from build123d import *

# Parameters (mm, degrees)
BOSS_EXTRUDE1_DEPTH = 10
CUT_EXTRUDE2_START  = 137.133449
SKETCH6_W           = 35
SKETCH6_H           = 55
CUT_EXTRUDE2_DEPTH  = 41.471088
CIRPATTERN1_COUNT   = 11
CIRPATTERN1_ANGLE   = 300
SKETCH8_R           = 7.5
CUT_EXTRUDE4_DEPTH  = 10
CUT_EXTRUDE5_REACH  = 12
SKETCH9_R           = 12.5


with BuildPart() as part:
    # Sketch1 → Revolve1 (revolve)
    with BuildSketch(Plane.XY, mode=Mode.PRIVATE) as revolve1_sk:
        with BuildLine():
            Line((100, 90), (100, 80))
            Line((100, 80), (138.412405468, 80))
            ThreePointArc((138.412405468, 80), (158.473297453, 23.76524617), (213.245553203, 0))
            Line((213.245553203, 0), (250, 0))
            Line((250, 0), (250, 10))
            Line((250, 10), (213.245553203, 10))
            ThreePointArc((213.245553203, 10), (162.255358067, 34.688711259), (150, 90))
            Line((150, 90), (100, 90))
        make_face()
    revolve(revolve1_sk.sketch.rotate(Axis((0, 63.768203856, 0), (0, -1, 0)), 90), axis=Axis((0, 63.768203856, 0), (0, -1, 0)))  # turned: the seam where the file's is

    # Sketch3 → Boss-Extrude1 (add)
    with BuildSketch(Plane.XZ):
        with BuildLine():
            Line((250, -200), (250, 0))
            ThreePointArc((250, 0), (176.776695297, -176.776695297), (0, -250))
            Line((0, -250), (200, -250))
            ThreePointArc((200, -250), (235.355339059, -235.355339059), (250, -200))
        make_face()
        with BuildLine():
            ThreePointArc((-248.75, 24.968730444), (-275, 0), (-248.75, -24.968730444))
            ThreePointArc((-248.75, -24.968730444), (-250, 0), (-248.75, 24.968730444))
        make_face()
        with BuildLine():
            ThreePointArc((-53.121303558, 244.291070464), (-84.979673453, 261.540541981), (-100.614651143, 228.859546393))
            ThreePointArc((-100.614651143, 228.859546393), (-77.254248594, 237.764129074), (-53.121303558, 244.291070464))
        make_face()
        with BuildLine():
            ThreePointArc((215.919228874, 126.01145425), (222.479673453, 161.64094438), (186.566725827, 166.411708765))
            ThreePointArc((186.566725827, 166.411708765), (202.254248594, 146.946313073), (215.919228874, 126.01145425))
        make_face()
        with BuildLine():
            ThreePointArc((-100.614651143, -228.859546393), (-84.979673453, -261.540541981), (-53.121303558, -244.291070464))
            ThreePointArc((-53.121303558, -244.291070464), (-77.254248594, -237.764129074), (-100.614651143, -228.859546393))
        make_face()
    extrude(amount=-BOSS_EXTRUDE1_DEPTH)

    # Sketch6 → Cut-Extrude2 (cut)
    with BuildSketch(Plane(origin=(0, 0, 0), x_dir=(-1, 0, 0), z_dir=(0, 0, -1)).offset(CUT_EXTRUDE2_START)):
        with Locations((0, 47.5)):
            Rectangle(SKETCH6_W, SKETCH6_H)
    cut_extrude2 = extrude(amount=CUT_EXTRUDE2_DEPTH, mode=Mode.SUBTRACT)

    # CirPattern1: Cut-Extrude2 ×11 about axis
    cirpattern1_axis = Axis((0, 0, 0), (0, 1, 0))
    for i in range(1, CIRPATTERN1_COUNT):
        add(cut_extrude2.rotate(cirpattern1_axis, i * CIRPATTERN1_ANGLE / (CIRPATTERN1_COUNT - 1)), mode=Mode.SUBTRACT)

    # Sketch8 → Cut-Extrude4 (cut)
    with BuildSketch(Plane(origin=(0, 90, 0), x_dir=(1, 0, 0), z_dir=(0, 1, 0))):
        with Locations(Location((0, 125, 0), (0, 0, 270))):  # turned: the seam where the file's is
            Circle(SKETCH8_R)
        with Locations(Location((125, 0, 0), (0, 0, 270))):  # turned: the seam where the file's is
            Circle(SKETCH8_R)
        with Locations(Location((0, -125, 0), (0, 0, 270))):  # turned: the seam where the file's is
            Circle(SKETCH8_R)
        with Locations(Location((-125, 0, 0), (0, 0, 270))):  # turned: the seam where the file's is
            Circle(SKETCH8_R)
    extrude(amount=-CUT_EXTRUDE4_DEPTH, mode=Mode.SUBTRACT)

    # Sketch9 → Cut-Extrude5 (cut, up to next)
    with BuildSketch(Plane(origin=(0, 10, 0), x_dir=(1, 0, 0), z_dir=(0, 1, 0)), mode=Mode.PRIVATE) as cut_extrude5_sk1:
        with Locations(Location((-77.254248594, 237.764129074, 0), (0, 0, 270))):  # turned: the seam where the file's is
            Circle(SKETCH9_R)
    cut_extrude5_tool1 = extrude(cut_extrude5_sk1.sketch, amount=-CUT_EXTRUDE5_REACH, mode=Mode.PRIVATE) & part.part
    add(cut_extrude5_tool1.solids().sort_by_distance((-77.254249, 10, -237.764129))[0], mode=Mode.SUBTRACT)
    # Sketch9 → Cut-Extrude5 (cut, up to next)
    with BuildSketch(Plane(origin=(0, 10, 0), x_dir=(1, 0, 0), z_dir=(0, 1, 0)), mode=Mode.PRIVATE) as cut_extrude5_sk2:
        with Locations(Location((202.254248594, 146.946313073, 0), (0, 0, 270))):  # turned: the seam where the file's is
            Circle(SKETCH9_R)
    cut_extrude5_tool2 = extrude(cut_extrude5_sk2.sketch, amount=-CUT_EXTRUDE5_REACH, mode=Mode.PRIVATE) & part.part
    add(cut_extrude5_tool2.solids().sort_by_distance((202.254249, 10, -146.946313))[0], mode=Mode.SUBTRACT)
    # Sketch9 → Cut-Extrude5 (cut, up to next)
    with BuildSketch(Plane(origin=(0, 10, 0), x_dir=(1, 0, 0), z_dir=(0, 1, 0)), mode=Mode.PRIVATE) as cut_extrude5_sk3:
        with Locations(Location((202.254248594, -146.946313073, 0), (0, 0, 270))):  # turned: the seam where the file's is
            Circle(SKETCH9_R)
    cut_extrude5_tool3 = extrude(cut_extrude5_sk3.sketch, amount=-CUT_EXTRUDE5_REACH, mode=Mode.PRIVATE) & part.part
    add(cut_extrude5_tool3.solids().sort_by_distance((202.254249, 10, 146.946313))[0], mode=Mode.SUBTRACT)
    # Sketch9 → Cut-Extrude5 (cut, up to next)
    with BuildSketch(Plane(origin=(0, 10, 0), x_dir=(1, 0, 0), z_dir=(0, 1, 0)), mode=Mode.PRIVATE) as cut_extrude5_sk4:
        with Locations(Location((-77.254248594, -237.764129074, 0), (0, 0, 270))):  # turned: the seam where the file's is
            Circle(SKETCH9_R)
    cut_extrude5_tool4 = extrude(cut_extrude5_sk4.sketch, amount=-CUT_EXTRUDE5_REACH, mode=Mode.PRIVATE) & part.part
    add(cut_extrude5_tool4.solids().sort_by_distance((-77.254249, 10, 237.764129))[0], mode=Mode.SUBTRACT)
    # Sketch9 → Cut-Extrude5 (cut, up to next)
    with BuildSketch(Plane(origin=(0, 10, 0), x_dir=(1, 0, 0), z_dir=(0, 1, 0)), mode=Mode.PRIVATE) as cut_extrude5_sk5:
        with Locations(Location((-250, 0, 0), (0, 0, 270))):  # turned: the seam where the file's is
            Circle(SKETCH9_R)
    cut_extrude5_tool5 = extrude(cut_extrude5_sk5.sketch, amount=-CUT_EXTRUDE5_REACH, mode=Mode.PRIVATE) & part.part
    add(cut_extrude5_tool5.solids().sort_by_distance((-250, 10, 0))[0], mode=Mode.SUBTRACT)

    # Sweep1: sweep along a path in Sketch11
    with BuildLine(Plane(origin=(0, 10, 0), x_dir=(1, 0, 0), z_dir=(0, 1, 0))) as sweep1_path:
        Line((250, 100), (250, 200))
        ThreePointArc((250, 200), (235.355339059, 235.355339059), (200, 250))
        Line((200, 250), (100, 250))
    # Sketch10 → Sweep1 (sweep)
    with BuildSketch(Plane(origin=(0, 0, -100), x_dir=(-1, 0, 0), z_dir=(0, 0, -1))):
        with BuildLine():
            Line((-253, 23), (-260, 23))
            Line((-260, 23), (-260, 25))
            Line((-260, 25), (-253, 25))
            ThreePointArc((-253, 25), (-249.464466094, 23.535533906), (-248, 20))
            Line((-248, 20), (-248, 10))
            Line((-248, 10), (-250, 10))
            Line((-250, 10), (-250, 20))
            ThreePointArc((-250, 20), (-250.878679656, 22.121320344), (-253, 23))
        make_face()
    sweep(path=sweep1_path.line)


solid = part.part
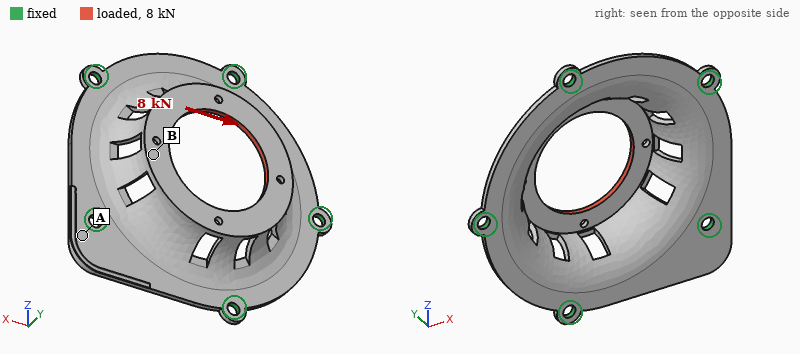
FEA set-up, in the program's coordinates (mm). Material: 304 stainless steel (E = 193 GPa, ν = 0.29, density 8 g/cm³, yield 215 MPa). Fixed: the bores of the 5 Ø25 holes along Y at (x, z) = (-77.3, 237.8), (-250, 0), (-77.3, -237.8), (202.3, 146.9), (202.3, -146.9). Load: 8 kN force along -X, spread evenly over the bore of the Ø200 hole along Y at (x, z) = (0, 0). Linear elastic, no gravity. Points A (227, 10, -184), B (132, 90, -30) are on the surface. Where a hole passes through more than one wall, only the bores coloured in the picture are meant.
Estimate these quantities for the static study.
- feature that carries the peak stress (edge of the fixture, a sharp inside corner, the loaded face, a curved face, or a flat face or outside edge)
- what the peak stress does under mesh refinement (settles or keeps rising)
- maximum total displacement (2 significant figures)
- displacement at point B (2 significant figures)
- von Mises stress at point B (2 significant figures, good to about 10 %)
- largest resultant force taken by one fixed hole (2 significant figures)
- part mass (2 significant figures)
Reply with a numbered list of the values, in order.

1. edge of the fixture
2. keeps rising
3. 31 µm
4. 25 µm
5. 4.3 MPa
6. 2.5 kN
7. 16 kg
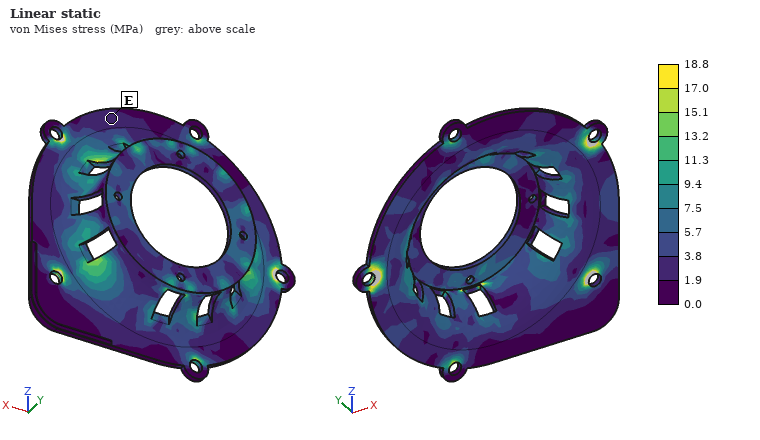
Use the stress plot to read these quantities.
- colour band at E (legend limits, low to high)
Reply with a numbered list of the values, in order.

1. 1.9 to 3.8 MPa
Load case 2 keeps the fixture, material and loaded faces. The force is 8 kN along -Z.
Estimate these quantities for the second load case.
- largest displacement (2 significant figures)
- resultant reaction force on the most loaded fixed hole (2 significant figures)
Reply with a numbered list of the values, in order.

1. 31 µm
2. 2.5 kN
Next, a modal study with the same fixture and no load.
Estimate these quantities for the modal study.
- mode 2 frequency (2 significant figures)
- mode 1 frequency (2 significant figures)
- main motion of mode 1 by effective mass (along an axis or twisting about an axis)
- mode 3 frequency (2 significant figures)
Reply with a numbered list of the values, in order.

1. 720 Hz
2. 650 Hz
3. along Y
4. 750 Hz
